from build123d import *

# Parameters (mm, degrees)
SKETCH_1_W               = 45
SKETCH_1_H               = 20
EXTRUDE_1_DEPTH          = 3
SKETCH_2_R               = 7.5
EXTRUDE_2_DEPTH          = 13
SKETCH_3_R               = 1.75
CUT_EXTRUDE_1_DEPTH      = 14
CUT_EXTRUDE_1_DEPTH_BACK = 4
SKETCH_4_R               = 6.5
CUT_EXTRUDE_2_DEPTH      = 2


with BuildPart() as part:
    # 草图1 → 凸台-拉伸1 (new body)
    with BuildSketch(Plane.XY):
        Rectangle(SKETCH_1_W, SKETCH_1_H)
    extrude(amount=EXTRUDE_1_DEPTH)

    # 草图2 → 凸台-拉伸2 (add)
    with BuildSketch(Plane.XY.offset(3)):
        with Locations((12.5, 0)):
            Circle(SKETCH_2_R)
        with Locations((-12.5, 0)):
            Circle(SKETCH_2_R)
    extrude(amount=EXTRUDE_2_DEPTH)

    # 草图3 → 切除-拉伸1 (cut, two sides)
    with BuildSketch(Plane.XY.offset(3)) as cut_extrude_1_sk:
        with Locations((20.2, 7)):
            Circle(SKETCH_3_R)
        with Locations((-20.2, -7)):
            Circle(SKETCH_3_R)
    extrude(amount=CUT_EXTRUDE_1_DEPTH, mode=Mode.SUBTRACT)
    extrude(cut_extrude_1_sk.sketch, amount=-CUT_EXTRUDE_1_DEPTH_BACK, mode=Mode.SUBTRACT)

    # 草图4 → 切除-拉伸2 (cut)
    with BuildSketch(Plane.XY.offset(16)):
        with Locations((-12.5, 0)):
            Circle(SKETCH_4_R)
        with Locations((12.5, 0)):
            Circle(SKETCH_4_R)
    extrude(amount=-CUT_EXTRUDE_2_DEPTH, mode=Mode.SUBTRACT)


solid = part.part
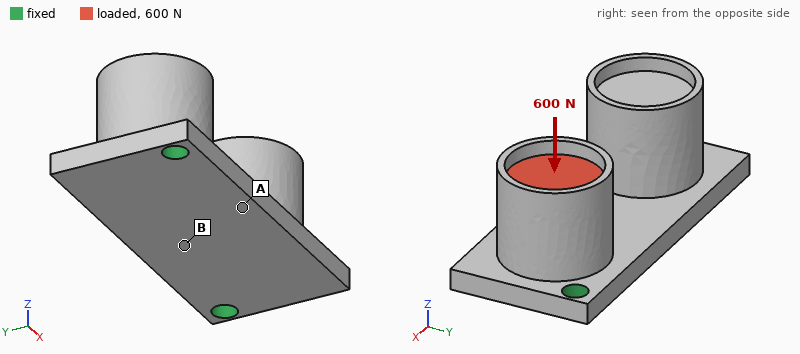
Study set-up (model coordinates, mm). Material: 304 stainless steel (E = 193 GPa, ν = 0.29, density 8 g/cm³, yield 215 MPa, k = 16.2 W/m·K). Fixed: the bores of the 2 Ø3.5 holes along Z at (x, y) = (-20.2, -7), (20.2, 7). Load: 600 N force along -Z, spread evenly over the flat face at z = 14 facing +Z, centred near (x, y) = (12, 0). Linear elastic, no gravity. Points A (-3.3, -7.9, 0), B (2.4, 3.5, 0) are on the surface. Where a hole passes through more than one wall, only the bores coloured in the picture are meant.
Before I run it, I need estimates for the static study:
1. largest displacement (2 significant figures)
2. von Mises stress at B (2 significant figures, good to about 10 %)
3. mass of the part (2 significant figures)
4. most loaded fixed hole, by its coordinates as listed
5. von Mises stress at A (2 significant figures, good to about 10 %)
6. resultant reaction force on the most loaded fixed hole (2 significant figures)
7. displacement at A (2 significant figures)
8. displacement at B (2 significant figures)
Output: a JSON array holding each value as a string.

["28 µm", "41 MPa", "54 g", "(20.2, 7)", "18 MPa", "490 N", "15 µm", "12 µm"]
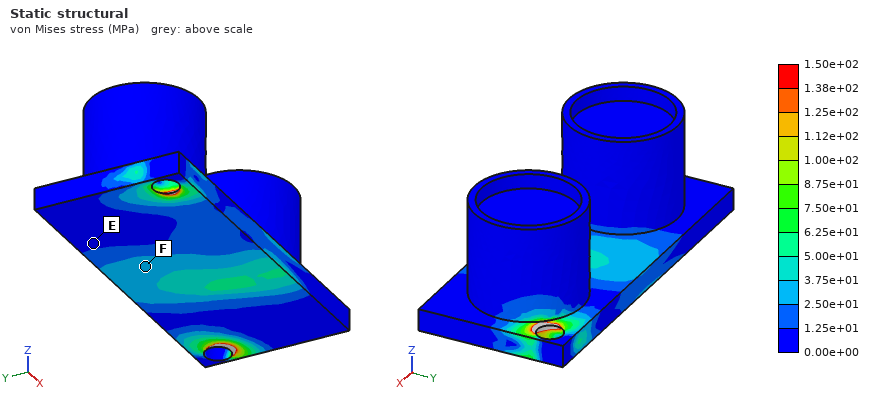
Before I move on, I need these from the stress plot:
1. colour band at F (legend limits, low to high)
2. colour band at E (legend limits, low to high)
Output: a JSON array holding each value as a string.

["2.50e+01 to 3.75e+01 MPa", "0.00e+00 to 1.25e+01 MPa"]
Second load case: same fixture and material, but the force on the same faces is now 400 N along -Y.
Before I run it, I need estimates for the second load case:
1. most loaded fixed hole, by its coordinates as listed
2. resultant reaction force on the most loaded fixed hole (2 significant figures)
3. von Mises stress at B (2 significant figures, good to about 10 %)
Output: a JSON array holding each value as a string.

["(20.2, 7)", "340 N", "31 MPa"]
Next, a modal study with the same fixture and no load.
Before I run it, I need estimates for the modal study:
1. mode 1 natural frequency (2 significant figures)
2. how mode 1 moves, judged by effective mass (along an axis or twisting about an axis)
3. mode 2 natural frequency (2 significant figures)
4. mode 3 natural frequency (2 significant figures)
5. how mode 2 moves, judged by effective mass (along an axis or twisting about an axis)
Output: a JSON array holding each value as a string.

["4400 Hz", "along Z", "4800 Hz", "7800 Hz", "along Y"]
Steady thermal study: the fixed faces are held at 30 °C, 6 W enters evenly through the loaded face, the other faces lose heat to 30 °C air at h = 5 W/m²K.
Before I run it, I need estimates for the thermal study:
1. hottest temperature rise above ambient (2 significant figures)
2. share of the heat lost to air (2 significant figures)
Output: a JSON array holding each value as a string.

["67 K", "8.3 %"]
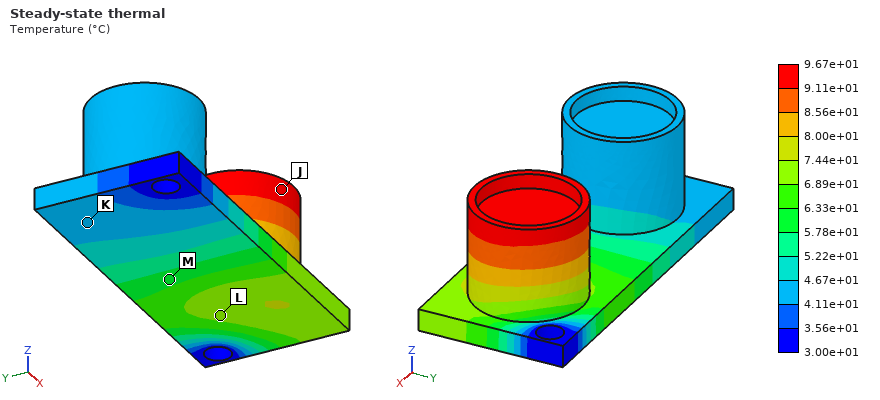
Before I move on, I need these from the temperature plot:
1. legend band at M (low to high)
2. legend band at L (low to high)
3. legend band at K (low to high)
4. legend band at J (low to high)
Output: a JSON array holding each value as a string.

["5.78e+01 to 6.33e+01 °C", "6.89e+01 to 7.44e+01 °C", "4.11e+01 to 4.67e+01 °C", "9.11e+01 to 9.67e+01 °C"]
